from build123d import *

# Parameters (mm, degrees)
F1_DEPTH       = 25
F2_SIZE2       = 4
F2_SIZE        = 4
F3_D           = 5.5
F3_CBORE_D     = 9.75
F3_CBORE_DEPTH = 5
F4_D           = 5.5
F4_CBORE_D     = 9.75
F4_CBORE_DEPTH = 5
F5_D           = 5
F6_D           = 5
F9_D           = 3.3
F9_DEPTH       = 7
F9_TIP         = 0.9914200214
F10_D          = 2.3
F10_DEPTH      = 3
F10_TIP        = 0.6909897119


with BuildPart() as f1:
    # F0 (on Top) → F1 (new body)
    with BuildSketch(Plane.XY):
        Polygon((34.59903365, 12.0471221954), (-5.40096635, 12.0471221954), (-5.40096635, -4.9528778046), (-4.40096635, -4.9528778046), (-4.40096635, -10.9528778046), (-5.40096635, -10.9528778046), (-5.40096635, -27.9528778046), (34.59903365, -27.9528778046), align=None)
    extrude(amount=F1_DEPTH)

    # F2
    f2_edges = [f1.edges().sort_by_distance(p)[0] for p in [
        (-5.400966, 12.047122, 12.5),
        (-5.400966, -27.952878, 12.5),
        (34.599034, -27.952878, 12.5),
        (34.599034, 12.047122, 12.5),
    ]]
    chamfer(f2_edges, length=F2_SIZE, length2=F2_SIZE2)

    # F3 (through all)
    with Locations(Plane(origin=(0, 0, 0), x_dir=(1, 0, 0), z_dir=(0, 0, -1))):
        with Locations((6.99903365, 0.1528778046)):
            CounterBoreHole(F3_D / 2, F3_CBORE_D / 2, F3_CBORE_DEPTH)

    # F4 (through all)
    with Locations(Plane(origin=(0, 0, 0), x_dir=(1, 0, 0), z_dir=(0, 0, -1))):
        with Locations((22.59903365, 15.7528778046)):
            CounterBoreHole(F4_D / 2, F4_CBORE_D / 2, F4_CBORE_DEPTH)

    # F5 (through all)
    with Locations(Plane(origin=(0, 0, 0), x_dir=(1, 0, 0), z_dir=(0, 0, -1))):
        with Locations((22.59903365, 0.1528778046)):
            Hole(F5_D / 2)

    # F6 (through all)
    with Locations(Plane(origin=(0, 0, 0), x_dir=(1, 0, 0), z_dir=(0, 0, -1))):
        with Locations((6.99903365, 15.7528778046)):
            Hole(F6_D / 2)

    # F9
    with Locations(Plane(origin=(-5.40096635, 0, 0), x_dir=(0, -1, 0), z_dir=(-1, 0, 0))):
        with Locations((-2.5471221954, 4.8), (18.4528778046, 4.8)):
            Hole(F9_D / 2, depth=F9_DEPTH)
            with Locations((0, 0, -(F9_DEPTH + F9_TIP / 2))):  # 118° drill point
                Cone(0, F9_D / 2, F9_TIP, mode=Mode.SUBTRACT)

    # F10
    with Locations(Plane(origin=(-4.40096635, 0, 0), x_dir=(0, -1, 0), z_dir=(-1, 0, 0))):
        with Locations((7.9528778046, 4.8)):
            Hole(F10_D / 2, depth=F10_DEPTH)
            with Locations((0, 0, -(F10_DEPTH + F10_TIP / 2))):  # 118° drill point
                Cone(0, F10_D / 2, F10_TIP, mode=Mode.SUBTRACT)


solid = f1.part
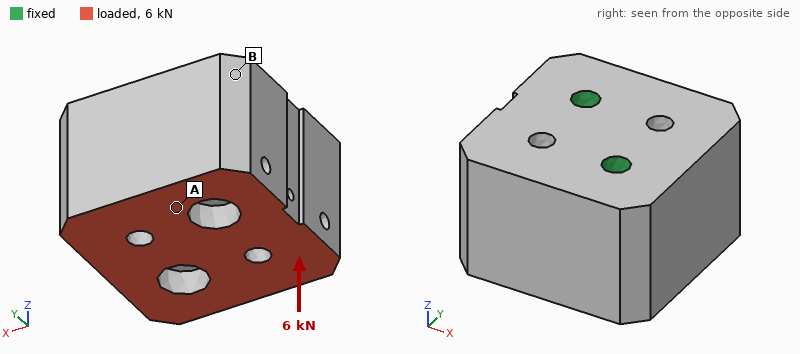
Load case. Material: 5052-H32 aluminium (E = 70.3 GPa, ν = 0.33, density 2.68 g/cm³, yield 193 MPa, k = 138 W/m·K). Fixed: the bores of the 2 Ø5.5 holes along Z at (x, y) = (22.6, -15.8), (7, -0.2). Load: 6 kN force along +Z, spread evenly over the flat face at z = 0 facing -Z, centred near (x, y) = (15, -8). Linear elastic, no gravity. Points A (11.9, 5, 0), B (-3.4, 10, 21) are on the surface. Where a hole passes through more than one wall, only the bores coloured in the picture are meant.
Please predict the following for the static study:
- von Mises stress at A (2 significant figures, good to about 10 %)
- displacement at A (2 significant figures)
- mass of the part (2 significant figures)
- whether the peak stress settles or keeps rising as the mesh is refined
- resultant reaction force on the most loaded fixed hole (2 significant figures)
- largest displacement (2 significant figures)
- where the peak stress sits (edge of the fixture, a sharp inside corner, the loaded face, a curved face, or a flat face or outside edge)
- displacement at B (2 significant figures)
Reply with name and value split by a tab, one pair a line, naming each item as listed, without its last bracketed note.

von Mises stress at A	6.4 MPa
displacement at A	2.2 µm
mass of the part	97 g
whether the peak stress settles or keeps rising as the mesh is refined	keeps rising
resultant reaction force on the most loaded fixed hole	3.0 kN
largest displacement	5.0 µm
where the peak stress sits	edge of the fixture
displacement at B	1.00 µm
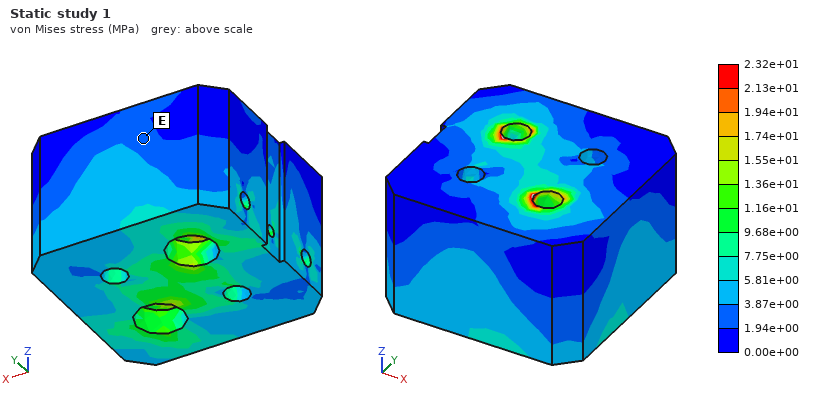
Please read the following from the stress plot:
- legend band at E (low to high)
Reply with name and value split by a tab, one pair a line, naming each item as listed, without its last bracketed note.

legend band at E	1.94e+00 to 3.87e+00 MPa
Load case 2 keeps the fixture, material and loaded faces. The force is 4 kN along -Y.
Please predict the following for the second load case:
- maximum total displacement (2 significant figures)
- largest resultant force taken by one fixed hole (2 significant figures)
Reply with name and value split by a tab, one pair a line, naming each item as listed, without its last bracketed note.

maximum total displacement	6.6 µm
largest resultant force taken by one fixed hole	2.2 kN
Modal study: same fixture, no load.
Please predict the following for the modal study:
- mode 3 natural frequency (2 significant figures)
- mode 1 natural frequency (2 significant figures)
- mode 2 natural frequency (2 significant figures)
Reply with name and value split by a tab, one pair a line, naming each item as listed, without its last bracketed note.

mode 3 natural frequency	27 kHz
mode 1 natural frequency	20 kHz
mode 2 natural frequency	26 kHz
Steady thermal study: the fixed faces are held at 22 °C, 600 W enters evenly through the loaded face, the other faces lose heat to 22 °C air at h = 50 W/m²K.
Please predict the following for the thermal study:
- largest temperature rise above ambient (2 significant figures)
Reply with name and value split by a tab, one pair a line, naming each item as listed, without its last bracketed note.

largest temperature rise above ambient	68 K
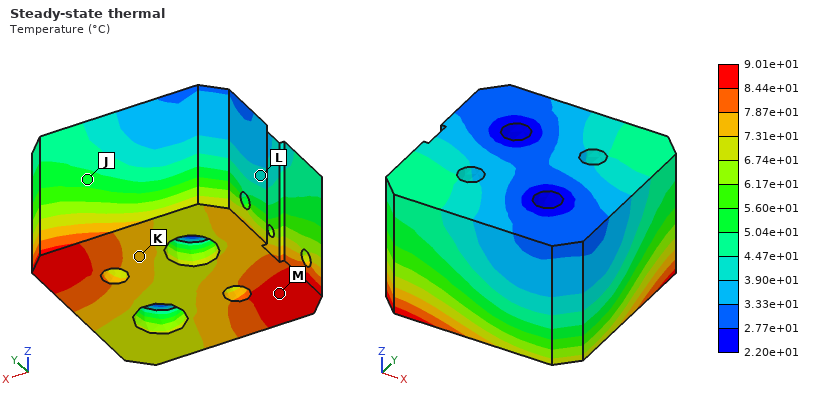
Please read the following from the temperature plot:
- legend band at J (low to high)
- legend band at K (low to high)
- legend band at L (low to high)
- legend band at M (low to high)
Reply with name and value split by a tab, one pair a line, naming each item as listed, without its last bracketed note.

legend band at J	5.04e+01 to 5.60e+01 °C
legend band at K	7.31e+01 to 7.87e+01 °C
legend band at L	3.90e+01 to 4.47e+01 °C
legend band at M	8.44e+01 to 9.01e+01 °C
